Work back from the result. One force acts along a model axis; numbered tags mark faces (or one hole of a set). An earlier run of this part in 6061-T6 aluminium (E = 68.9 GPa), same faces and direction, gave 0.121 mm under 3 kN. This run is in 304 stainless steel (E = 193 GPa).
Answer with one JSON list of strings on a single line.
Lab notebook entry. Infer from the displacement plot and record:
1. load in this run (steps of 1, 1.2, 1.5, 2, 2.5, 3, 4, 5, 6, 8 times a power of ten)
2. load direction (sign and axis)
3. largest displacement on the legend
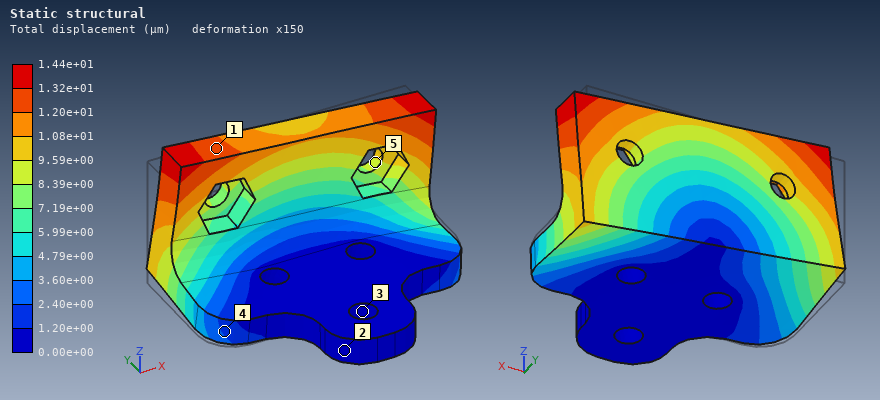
["1 kN", "+X", "1.44e+01 µm"]
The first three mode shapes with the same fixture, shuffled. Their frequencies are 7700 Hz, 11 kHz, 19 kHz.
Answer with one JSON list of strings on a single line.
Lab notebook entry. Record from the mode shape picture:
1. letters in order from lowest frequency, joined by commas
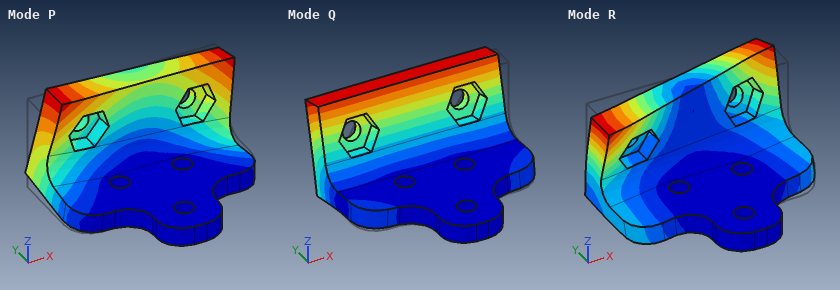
["Q, P, R"]
